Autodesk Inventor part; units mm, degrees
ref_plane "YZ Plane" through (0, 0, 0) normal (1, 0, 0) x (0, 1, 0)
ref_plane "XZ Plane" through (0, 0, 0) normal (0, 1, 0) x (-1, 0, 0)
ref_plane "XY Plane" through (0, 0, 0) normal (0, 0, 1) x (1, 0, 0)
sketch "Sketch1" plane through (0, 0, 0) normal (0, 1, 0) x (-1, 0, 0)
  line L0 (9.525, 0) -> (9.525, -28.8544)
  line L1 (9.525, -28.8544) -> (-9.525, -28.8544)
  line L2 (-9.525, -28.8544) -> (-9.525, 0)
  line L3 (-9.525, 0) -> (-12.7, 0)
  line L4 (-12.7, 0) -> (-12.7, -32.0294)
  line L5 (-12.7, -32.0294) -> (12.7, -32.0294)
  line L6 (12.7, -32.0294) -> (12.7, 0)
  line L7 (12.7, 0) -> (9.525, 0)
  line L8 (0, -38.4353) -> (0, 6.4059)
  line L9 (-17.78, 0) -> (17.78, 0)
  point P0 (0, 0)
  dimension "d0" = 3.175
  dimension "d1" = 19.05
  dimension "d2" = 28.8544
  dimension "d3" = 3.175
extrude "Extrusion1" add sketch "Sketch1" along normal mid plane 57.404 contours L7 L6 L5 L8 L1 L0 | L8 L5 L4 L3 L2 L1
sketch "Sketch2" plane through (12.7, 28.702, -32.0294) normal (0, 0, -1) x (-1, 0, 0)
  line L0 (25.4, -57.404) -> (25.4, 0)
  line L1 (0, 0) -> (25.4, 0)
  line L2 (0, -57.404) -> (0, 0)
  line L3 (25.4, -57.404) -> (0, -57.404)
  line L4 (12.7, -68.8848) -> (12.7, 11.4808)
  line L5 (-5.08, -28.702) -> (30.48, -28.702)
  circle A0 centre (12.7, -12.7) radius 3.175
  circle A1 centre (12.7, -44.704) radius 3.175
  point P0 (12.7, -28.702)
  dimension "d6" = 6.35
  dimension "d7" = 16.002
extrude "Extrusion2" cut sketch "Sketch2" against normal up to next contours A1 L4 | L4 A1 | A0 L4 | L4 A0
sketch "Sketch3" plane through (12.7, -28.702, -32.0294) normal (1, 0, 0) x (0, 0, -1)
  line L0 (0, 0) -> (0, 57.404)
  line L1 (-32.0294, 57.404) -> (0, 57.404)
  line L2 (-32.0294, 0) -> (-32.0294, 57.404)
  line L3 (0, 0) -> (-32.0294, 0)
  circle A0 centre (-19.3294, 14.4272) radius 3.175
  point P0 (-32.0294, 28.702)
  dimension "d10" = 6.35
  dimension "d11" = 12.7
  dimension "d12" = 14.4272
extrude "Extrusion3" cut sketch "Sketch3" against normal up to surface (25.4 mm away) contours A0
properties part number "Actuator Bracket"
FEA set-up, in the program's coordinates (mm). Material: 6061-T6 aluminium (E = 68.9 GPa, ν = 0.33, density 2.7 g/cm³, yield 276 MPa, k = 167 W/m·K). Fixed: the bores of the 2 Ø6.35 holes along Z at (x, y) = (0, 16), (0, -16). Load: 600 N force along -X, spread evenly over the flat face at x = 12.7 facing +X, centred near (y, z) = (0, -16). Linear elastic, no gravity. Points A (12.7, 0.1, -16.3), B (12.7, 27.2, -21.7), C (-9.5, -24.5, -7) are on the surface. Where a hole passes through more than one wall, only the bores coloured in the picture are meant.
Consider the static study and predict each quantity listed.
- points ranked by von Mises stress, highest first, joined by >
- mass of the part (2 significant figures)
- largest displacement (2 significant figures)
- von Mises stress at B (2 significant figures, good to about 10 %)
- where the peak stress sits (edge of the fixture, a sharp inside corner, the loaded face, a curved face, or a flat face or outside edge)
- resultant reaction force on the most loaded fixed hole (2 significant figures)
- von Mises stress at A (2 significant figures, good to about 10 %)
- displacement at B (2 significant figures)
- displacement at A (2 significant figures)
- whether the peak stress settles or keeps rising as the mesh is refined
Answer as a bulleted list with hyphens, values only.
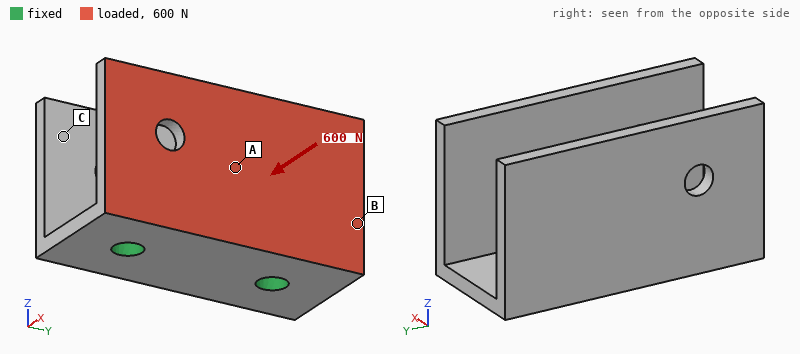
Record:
- B > A > C
- 40 g
- 0.39 mm
- 46 MPa
- edge of the fixture
- 310 N
- 24 MPa
- 0.10 mm
- 0.16 mm
- keeps rising
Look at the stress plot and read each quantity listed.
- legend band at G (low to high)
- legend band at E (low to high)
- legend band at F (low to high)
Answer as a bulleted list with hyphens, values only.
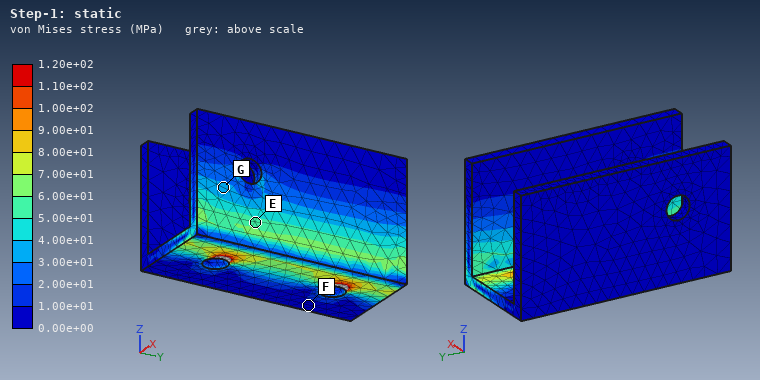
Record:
- 3.00e+01 to 4.00e+01 MPa
- 5.00e+01 to 6.00e+01 MPa
- 0.00e+00 to 1.00e+01 MPa
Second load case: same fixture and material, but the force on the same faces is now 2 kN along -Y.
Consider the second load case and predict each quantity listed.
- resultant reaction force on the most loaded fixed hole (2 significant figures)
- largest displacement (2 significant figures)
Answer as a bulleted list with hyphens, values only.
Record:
- 1.4 kN
- 0.11 mm
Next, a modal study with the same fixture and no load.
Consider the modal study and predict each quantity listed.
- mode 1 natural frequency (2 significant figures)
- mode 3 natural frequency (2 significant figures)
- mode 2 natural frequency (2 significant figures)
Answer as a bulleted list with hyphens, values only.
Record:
- 1900 Hz
- 3400 Hz
- 2000 Hz
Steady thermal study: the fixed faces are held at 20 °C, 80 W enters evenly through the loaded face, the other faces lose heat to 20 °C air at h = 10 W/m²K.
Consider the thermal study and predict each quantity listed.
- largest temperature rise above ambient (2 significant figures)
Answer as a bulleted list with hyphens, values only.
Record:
- 67 K
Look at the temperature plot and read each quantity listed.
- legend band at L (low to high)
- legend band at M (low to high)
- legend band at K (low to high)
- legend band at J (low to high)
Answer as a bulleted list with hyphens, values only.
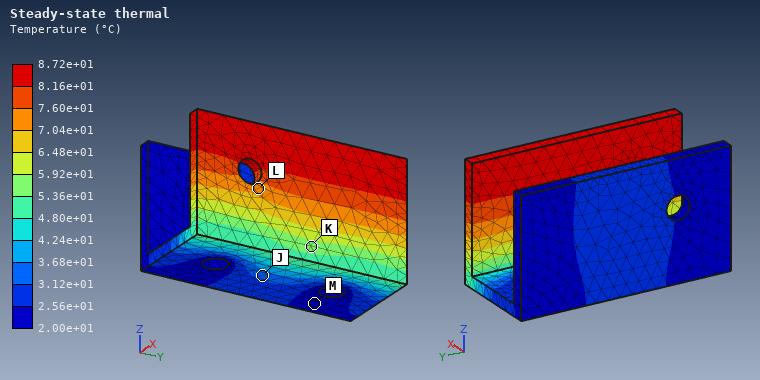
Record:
- 7.04e+01 to 7.60e+01 °C
- 2.00e+01 to 2.56e+01 °C
- 5.36e+01 to 5.92e+01 °C
- 3.12e+01 to 3.68e+01 °C
